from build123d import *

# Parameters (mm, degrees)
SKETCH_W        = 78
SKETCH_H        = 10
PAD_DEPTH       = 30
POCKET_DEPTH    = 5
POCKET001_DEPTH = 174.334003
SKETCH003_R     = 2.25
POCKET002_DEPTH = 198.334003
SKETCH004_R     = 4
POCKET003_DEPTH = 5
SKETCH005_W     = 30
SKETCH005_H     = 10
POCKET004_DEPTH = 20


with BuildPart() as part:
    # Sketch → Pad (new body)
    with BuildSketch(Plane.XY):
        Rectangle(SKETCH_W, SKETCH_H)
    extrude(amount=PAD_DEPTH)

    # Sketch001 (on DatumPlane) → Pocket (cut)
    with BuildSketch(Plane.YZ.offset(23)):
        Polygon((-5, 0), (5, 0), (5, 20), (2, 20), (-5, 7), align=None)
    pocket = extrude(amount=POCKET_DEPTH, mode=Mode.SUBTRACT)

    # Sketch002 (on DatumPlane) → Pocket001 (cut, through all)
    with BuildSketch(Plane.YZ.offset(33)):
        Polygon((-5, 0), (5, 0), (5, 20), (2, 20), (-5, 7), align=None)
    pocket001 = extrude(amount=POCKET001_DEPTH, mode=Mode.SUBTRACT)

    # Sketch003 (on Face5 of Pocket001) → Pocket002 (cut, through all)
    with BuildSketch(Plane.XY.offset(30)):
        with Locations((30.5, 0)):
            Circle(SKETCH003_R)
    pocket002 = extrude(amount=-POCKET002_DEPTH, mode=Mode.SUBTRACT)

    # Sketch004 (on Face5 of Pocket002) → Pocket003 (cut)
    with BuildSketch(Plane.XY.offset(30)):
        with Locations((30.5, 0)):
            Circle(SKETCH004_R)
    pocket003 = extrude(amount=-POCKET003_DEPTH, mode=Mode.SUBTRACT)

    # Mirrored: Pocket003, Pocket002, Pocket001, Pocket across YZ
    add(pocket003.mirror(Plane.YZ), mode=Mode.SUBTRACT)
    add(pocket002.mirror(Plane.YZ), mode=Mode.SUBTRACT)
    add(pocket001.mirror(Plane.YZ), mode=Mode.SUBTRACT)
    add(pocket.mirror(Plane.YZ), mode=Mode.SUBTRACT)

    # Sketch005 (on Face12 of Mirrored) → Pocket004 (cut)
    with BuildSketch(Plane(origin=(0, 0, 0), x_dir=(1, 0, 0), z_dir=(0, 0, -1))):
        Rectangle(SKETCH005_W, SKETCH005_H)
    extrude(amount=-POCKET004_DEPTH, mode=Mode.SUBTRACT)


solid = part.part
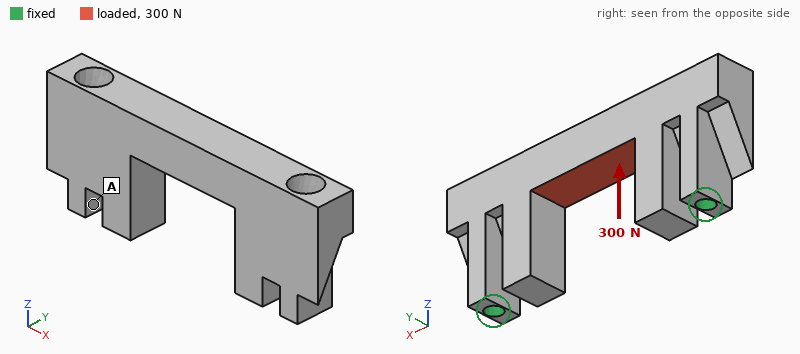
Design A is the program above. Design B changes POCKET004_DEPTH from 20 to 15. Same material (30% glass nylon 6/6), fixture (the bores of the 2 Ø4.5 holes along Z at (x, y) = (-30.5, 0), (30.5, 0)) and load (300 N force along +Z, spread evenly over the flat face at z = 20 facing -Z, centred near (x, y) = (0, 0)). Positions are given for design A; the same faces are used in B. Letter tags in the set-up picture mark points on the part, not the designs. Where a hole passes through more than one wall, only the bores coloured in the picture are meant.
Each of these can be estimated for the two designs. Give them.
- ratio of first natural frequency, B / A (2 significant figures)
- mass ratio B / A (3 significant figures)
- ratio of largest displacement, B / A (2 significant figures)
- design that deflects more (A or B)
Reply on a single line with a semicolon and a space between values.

0.97; 1.12; 0.72; A
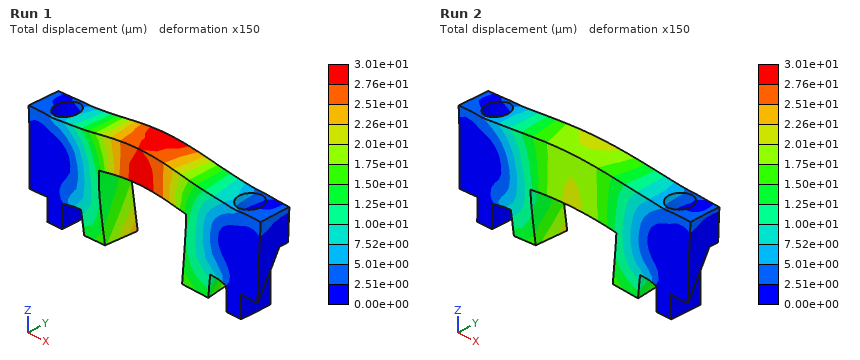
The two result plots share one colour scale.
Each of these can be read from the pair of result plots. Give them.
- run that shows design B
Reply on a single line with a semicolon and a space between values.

Run 2
